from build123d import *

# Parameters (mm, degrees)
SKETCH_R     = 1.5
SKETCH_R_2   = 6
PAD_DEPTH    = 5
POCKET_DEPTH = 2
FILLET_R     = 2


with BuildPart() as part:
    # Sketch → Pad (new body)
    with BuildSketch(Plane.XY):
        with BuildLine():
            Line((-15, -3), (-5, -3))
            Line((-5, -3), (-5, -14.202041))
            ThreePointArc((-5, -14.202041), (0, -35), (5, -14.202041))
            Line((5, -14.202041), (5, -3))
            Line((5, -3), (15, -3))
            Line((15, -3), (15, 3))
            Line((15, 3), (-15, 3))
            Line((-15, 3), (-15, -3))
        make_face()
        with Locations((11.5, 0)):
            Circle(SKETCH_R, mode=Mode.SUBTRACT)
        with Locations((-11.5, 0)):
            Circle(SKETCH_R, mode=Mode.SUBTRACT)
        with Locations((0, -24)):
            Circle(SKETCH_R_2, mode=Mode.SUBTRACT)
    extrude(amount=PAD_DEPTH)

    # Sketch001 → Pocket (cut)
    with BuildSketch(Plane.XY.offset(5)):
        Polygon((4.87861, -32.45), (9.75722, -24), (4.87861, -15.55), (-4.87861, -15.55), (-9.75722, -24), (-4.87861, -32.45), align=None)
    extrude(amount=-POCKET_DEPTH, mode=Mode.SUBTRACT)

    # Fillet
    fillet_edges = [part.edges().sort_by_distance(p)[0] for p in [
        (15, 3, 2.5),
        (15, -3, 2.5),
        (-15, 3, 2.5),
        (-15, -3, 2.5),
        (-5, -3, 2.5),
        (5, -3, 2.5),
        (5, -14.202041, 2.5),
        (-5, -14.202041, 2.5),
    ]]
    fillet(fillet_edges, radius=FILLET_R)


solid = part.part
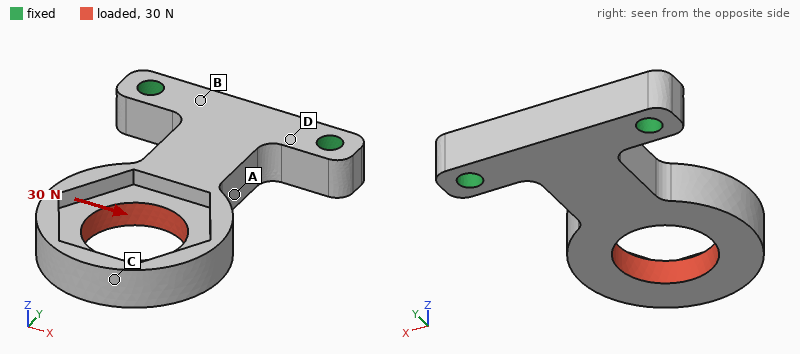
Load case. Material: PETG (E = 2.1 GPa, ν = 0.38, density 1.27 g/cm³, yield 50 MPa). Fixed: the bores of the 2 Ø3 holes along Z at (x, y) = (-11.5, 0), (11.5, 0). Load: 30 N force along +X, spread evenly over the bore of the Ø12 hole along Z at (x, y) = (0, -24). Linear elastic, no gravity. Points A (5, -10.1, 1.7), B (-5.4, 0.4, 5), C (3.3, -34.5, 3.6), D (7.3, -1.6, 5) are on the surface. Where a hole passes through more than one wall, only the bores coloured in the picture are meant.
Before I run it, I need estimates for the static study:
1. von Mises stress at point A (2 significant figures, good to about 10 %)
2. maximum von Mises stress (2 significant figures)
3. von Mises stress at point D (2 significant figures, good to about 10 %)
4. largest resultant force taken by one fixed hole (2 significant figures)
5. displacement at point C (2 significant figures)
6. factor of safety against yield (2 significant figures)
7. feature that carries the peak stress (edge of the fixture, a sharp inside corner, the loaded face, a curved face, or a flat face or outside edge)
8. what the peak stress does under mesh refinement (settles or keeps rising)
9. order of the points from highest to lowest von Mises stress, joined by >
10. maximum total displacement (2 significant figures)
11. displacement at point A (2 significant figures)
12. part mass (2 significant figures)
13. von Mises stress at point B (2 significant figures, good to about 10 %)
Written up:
5.2 MPa
12 MPa
4.1 MPa
42 N
0.38 mm
4.0
a curved face
settles
A > D > B > C
0.39 mm
0.059 mm
3.1 g
1.9 MPa
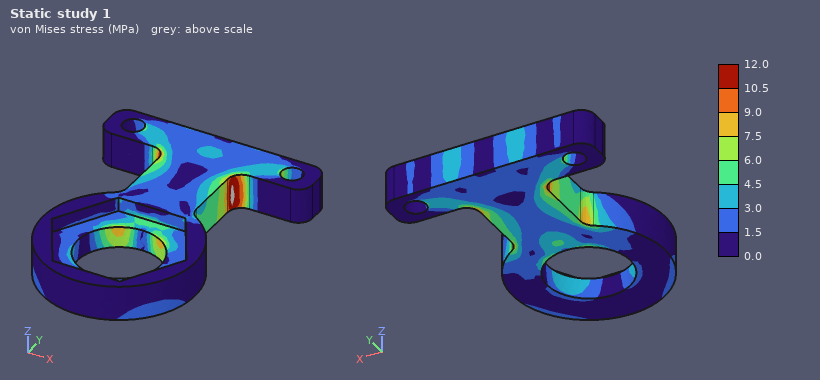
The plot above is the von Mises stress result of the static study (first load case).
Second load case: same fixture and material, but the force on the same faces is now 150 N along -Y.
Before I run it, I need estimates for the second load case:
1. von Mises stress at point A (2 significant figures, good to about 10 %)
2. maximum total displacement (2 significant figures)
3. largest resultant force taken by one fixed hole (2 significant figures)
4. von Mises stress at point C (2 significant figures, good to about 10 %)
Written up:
4.4 MPa
0.49 mm
81 N
2.9 MPa
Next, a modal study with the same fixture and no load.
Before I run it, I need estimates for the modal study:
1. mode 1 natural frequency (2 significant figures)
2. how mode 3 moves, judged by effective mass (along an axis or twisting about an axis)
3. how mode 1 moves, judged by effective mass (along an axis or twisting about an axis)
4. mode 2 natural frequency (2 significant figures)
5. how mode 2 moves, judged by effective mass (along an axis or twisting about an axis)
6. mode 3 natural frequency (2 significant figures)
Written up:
620 Hz
twisting about Y
along Z
1300 Hz
along X
2000 Hz
